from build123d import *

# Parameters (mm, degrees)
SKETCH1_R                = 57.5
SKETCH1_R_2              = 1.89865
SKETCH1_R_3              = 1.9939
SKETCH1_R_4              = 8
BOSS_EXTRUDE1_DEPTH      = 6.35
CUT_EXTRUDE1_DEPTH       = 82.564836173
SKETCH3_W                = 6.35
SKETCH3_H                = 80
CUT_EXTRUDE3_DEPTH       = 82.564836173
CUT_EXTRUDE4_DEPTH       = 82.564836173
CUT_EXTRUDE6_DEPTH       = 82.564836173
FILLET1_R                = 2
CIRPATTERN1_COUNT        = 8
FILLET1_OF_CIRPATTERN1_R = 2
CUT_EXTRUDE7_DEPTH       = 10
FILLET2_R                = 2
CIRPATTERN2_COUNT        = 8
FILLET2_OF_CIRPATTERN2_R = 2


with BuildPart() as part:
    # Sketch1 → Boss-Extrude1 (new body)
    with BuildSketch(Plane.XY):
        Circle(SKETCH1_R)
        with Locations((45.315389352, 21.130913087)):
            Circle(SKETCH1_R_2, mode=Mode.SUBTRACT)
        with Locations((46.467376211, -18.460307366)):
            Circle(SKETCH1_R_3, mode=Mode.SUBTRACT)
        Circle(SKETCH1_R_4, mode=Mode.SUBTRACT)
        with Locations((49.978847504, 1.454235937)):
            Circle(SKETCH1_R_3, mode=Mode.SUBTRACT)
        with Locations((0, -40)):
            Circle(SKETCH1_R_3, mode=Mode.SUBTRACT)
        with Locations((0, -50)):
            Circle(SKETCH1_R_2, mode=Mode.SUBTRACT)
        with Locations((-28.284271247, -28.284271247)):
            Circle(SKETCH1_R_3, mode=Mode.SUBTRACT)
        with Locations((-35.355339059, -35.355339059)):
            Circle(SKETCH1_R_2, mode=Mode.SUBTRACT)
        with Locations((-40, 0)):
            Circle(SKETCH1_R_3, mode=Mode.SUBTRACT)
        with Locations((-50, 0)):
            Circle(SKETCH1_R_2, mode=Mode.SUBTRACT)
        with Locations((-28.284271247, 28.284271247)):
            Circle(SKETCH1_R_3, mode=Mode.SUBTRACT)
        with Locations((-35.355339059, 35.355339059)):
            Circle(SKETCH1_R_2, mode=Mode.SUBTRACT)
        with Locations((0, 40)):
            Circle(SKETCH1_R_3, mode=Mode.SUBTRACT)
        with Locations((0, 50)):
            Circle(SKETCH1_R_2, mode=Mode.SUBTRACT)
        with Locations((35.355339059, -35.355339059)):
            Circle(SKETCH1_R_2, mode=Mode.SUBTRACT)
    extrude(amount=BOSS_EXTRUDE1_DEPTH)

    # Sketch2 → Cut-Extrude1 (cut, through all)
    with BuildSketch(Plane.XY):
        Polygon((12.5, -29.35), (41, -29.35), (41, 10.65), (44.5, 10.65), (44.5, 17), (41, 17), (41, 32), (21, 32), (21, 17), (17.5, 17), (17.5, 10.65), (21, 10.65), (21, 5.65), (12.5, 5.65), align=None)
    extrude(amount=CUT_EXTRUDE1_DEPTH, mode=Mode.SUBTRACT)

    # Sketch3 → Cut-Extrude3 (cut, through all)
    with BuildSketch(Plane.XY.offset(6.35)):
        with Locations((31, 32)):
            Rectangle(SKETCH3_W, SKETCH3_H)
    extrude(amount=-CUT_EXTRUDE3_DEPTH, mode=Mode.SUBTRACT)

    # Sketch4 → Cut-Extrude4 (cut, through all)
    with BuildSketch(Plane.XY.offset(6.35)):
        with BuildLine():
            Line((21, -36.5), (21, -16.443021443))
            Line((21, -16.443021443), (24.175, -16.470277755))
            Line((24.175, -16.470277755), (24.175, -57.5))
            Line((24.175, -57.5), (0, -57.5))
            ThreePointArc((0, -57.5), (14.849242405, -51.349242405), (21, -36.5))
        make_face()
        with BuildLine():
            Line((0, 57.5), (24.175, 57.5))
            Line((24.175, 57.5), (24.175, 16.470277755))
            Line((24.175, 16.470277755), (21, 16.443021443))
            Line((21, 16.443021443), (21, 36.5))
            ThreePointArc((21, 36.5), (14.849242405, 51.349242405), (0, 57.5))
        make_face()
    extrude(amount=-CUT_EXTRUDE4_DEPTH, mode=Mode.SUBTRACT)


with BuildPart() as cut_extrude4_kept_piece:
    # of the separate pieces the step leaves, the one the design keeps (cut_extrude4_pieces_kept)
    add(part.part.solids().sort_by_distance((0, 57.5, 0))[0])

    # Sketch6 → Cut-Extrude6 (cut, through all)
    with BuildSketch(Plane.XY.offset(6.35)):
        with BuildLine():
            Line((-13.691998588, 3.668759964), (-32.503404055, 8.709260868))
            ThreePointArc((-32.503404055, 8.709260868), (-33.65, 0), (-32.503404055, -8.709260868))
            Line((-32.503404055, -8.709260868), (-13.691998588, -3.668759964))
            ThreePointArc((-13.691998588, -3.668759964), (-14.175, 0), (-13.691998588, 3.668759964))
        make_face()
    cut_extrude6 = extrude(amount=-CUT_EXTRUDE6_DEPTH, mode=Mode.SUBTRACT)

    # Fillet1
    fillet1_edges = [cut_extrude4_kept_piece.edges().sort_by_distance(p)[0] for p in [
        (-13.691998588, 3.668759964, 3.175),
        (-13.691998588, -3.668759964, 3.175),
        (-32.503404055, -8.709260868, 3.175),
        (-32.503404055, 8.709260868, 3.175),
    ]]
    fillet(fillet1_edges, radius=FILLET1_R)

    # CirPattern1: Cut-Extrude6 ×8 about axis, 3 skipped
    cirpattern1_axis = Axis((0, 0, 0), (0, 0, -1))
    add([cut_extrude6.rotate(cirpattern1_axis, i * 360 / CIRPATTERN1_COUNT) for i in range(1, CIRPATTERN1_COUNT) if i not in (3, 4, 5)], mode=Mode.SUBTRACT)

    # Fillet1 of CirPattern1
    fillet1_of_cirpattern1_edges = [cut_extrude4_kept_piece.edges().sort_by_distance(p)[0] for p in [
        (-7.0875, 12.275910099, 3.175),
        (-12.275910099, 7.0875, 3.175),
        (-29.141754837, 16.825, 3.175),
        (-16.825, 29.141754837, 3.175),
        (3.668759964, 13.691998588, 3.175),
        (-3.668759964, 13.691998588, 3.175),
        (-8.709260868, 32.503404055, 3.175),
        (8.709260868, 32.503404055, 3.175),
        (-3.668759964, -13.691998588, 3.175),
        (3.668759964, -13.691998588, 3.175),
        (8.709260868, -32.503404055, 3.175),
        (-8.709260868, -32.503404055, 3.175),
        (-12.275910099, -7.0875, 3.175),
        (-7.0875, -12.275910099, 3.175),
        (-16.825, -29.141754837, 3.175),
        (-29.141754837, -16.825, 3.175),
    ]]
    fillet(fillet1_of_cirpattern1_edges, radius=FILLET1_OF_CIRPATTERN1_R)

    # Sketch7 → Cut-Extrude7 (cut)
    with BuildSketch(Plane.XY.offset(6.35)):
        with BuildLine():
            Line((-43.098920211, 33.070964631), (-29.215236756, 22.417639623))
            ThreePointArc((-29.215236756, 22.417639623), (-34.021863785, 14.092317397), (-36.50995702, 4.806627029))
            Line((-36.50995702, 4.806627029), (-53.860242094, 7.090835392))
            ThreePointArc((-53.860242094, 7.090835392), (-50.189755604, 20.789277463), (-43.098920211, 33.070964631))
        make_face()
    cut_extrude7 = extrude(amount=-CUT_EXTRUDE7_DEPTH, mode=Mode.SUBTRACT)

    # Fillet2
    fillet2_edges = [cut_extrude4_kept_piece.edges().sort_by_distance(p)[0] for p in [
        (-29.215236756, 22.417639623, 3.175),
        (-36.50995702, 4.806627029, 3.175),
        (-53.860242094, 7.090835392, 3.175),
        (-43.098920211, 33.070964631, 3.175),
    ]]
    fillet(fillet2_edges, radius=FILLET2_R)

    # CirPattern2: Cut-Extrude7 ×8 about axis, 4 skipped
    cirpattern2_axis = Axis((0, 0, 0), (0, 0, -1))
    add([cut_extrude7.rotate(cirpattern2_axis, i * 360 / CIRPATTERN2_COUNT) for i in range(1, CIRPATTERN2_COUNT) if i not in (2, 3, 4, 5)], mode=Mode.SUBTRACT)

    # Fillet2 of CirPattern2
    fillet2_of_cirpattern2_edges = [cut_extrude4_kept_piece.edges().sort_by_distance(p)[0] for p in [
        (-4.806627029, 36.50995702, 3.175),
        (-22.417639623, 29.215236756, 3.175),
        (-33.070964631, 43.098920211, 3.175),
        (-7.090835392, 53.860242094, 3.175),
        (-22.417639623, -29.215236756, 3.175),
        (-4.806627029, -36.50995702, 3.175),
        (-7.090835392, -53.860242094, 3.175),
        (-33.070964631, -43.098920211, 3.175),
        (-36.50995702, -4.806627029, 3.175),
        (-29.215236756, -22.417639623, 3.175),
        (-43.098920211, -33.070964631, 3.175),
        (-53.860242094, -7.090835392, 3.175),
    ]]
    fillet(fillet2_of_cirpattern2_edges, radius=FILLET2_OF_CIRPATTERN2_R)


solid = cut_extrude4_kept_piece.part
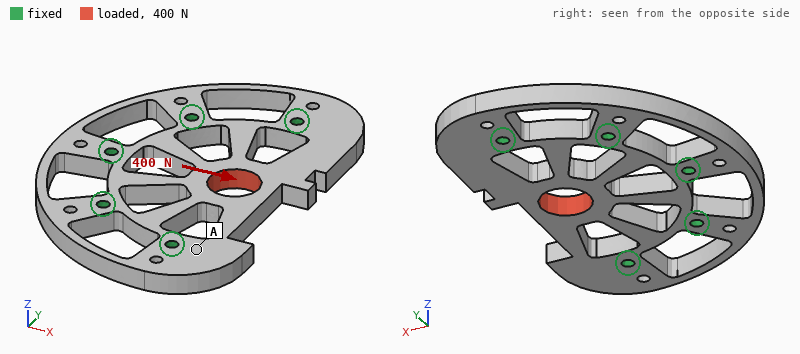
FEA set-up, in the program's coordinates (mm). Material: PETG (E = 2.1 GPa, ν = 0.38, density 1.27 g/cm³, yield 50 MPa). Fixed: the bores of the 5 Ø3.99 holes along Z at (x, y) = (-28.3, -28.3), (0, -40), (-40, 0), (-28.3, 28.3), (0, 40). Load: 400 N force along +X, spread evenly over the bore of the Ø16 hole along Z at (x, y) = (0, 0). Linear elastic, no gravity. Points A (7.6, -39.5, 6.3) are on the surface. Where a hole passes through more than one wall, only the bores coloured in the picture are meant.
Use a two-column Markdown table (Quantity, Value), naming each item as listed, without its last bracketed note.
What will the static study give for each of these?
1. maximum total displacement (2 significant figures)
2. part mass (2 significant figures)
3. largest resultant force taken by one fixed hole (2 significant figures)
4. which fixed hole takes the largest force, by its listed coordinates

| Quantity | Value |
|---|---|
| maximum total displacement | 0.18 mm |
| part mass | 32 g |
| largest resultant force taken by one fixed hole | 150 N |
| which fixed hole takes the largest force, by its listed coordinates | (-40, 0) |
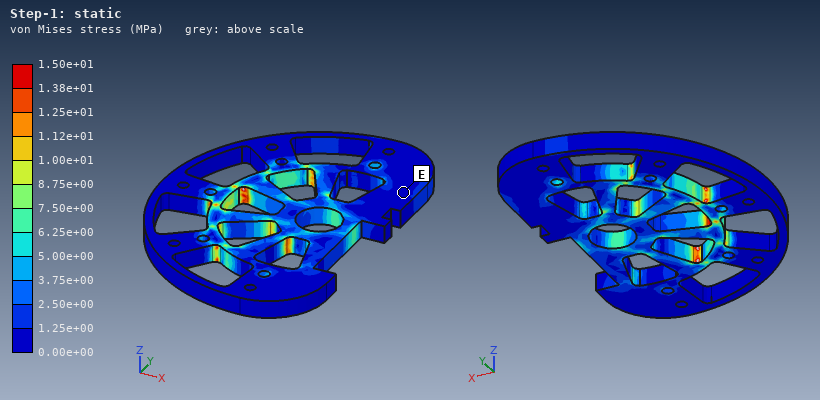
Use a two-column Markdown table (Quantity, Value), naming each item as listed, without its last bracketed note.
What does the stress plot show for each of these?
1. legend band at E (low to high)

| Quantity | Value |
|---|---|
| legend band at E | 0.00e+00 to 1.25e+00 MPa |
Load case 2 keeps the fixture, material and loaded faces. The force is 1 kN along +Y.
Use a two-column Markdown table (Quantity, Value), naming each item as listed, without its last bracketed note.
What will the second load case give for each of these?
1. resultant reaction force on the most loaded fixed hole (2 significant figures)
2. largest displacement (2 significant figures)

| Quantity | Value |
|---|---|
| resultant reaction force on the most loaded fixed hole | 380 N |
| largest displacement | 0.21 mm |
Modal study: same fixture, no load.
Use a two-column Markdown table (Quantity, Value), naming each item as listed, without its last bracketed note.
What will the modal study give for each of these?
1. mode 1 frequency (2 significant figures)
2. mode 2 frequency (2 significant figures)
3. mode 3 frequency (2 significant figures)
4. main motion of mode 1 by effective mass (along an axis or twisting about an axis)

| Quantity | Value |
|---|---|
| mode 1 frequency | 1000 Hz |
| mode 2 frequency | 2000 Hz |
| mode 3 frequency | 2500 Hz |
| main motion of mode 1 by effective mass | along Z |
